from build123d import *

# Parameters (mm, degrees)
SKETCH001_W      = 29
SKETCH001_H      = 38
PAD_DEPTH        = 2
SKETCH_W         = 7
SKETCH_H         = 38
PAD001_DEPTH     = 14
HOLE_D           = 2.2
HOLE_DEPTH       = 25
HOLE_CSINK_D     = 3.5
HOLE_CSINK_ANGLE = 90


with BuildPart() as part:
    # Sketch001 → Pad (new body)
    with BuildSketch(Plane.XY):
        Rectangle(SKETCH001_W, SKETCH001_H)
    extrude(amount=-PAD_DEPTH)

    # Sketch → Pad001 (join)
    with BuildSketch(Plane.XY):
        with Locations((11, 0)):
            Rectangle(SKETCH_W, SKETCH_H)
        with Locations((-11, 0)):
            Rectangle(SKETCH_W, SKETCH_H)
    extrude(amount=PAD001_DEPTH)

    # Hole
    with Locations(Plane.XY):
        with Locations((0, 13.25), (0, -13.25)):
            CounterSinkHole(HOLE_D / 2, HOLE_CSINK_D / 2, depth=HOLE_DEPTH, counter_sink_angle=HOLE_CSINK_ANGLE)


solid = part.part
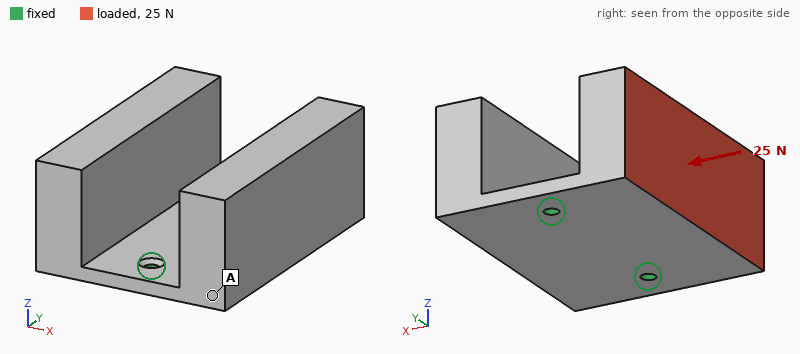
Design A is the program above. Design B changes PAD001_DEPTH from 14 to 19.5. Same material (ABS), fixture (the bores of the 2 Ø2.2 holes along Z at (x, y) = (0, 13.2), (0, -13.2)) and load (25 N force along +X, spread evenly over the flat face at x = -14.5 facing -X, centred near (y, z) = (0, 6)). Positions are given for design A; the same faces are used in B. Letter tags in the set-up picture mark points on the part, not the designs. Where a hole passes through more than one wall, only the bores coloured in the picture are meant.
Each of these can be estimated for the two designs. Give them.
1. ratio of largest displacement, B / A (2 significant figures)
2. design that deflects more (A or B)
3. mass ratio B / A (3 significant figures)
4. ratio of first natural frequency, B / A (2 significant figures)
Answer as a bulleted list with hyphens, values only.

- 1.7
- B
- 1.30
- 0.73
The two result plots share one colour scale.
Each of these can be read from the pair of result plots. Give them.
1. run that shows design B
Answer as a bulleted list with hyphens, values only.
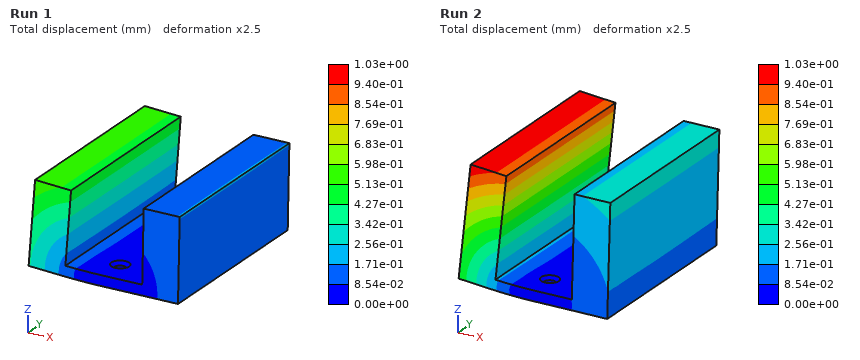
- Run 2
